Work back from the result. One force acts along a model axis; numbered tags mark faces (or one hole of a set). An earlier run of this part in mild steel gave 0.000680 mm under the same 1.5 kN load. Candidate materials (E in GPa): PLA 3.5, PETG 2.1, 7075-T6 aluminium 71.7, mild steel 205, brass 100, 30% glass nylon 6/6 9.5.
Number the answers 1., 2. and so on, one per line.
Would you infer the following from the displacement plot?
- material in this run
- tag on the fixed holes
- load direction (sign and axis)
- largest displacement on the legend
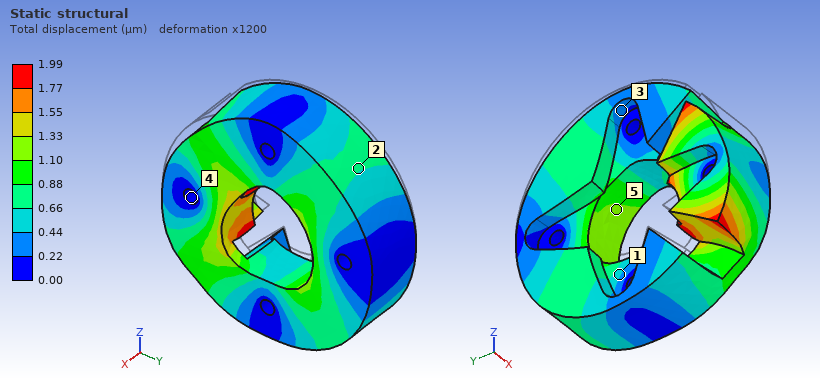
1. 7075-T6 aluminium
2. 4
3. -Z
4. 1.99 µm
